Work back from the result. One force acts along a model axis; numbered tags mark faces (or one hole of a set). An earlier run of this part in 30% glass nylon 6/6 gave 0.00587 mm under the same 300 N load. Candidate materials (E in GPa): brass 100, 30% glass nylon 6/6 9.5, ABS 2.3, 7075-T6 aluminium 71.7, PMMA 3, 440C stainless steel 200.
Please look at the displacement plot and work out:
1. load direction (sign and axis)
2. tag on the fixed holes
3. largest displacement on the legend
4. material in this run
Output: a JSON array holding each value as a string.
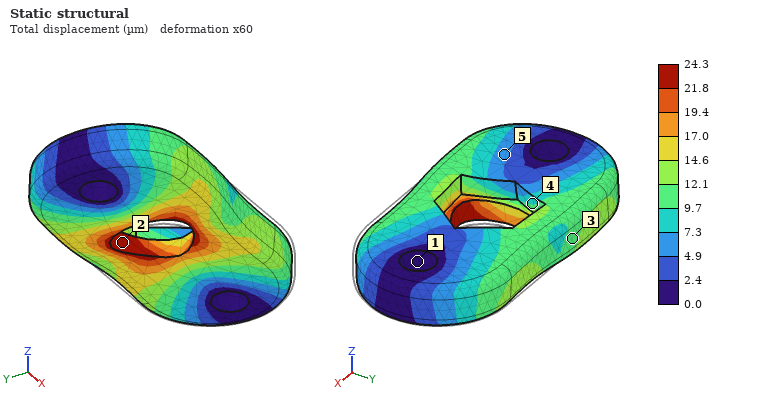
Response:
["-X", "1", "24.3 µm", "ABS"]
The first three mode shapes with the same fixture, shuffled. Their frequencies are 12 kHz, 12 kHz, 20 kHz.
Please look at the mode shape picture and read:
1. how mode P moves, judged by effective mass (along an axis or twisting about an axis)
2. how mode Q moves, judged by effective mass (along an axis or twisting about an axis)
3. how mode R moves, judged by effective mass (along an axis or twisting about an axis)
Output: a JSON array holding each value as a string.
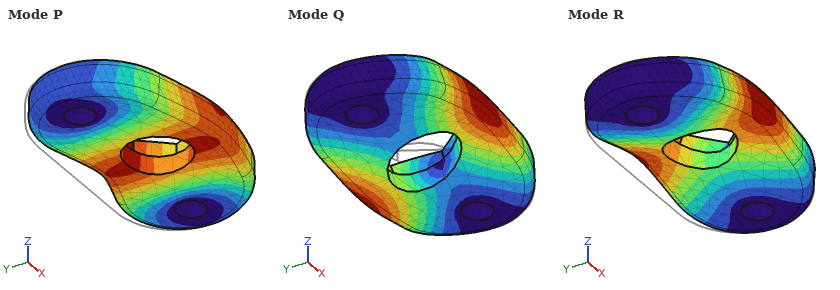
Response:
["along Y", "twisting about X", "along Z"]
